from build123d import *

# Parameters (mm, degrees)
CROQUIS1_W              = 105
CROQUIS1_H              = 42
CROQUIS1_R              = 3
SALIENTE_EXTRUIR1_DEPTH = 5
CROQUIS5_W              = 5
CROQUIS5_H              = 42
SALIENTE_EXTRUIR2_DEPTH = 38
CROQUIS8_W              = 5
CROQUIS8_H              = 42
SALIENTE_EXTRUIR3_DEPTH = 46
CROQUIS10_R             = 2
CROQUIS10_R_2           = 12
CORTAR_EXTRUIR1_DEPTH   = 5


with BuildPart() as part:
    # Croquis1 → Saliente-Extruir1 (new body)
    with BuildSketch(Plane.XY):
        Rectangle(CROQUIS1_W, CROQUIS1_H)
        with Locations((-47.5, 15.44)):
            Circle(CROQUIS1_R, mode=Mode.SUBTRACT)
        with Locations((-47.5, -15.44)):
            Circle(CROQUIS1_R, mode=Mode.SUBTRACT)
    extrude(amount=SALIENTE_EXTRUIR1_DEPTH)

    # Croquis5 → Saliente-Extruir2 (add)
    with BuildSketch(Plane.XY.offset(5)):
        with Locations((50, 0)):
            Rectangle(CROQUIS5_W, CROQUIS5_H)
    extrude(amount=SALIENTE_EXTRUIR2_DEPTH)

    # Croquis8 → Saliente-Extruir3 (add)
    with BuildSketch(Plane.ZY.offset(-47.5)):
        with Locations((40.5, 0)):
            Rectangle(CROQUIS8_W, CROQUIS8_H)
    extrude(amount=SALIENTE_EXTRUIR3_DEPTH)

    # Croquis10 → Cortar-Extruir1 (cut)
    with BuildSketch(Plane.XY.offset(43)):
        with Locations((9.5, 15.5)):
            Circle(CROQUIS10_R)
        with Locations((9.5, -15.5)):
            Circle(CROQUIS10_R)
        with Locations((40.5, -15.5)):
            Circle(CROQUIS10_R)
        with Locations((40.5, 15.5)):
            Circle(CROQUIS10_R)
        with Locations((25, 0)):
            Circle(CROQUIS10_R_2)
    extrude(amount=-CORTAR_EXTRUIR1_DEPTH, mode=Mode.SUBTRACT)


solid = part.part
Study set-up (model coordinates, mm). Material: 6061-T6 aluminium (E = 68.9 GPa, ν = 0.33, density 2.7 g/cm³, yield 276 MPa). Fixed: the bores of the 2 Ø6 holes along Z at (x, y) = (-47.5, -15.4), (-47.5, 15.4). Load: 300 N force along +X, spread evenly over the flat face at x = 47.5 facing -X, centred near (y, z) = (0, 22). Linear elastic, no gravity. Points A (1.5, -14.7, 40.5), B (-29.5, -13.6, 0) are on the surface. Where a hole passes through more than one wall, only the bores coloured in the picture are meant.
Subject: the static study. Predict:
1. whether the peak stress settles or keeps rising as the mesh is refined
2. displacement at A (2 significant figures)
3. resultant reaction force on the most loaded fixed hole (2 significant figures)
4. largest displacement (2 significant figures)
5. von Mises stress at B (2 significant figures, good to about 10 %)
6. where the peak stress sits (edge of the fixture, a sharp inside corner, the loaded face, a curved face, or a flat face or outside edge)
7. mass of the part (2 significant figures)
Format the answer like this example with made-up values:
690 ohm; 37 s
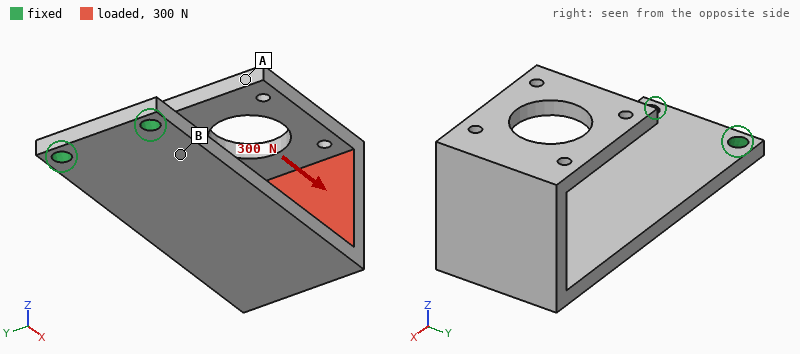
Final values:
keeps rising; 0.74 mm; 150 N; 1.2 mm; 30 MPa; edge of the fixture; 100 g
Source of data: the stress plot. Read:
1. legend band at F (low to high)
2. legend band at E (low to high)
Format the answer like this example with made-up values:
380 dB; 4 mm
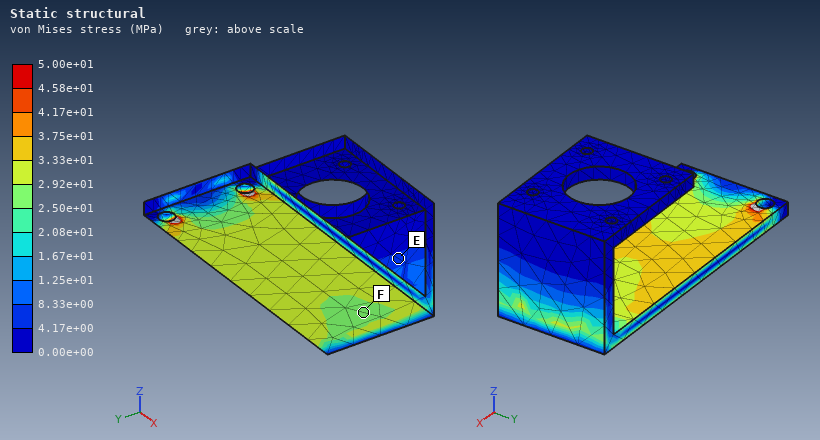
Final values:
2.50e+01 to 2.92e+01 MPa; 4.17e+00 to 8.33e+00 MPa
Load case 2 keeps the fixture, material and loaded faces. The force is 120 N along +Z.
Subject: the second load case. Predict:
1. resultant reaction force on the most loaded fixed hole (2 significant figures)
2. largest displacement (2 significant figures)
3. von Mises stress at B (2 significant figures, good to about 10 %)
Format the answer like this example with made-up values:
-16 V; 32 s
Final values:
60 N; 1.4 mm; 51 MPa
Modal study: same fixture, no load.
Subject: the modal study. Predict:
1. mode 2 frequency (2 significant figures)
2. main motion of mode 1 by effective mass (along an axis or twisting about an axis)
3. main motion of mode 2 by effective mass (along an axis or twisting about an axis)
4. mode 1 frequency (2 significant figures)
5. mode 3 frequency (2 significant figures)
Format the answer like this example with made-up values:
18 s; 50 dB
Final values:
490 Hz; along Z; along Y; 220 Hz; 570 Hz
